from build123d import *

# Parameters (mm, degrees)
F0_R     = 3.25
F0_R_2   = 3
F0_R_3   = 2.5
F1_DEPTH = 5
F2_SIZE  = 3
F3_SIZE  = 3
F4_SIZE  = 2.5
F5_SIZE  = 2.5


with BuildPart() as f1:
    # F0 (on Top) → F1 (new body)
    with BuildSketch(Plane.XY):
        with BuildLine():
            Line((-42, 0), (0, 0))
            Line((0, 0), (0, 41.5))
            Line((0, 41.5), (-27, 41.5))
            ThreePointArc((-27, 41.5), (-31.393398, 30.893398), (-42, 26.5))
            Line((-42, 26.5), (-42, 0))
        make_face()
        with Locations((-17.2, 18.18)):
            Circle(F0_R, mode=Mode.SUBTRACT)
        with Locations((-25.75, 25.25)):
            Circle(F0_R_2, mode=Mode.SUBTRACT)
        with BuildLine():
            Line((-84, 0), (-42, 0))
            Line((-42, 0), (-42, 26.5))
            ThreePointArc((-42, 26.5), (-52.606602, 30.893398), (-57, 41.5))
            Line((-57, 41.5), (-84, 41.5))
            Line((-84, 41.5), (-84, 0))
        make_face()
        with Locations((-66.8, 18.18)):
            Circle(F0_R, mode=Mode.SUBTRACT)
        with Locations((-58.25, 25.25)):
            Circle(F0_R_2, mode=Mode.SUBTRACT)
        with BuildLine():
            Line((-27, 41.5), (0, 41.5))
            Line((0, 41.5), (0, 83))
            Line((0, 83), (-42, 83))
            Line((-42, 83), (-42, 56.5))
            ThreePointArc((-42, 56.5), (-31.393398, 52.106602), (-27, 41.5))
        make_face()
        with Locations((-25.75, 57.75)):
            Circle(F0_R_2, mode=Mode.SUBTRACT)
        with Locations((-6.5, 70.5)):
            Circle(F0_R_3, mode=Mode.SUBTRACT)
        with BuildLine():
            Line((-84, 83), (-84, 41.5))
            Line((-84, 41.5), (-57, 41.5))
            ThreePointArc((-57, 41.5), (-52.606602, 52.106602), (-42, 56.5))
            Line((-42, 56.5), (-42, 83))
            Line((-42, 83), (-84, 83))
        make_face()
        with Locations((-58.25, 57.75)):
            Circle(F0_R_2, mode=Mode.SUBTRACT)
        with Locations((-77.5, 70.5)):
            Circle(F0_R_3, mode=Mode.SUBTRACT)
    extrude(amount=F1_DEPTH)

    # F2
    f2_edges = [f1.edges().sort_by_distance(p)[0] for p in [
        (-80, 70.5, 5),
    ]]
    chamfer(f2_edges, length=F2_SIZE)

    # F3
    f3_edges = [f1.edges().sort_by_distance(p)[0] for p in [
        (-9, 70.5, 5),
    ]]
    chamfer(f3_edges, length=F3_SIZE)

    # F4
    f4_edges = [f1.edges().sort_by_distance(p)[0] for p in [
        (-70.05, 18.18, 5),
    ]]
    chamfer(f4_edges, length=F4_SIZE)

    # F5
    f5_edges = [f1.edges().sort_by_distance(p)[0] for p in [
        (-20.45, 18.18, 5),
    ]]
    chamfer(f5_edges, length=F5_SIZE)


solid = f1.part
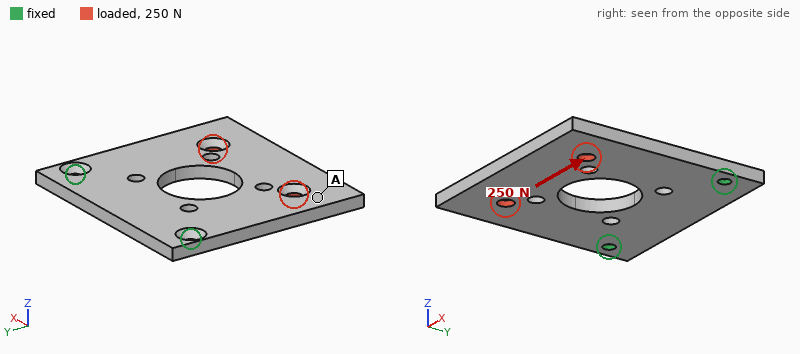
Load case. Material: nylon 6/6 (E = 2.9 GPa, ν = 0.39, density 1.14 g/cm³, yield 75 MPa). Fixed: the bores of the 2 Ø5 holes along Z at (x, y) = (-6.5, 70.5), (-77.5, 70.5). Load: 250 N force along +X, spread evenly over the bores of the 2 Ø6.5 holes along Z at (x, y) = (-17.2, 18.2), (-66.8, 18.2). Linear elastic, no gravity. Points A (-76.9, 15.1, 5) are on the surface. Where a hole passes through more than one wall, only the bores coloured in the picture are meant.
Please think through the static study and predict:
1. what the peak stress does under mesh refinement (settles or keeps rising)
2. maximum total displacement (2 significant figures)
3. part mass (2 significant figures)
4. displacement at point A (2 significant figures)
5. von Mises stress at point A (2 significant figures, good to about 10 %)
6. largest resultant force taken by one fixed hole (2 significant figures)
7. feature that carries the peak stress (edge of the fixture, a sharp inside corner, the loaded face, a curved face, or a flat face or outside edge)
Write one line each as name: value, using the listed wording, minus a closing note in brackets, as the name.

what the peak stress does under mesh refinement: keeps rising
maximum total displacement: 0.31 mm
part mass: 34 g
displacement at point A: 0.22 mm
von Mises stress at point A: 1.3 MPa
largest resultant force taken by one fixed hole: 220 N
feature that carries the peak stress: edge of the fixture
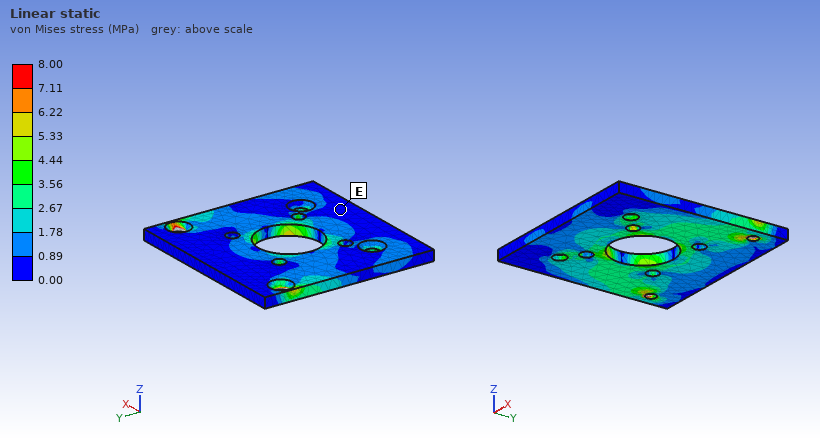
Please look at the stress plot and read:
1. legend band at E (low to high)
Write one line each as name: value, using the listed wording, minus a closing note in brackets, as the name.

legend band at E: 0.00 to 0.89 MPa
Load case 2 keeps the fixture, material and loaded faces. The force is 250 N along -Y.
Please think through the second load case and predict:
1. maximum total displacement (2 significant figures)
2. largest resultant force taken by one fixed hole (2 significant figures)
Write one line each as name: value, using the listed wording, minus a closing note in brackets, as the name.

maximum total displacement: 0.37 mm
largest resultant force taken by one fixed hole: 130 N
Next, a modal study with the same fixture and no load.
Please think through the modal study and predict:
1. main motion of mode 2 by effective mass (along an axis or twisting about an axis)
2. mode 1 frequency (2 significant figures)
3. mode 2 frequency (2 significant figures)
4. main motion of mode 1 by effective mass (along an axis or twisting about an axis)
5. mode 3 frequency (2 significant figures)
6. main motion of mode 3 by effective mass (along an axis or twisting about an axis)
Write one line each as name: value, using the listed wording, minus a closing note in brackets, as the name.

main motion of mode 2 by effective mass: twisting about Y
mode 1 frequency: 170 Hz
mode 2 frequency: 460 Hz
main motion of mode 1 by effective mass: along Z
mode 3 frequency: 1100 Hz
main motion of mode 3 by effective mass: along Z
